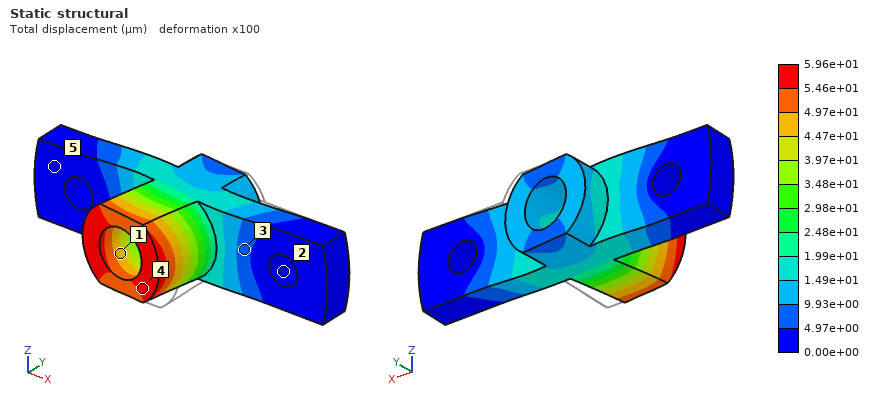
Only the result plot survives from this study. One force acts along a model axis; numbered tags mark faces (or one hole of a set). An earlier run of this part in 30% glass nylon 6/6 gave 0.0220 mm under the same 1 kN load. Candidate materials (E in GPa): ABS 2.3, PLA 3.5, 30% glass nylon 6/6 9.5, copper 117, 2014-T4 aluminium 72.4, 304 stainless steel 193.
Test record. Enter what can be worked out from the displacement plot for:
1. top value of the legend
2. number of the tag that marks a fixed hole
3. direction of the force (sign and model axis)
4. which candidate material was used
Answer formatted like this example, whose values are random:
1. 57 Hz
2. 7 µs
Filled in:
1. 5.96e+01 µm
2. 2
3. -X
4. PLA
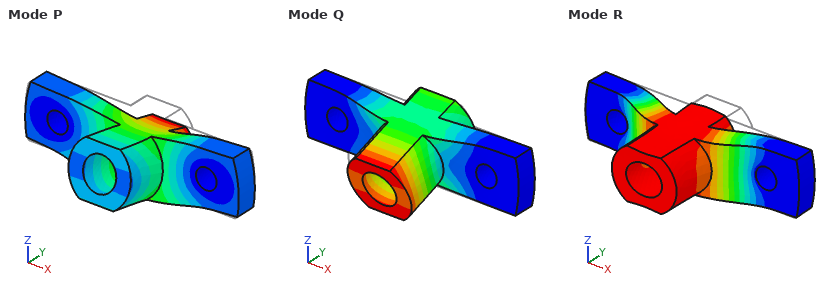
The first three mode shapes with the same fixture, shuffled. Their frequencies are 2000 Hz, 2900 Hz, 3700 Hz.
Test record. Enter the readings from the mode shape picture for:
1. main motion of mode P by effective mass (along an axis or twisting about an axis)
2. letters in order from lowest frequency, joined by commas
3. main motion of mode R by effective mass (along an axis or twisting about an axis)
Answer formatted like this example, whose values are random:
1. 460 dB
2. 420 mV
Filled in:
1. along Z
2. Q, R, P
3. along Y
